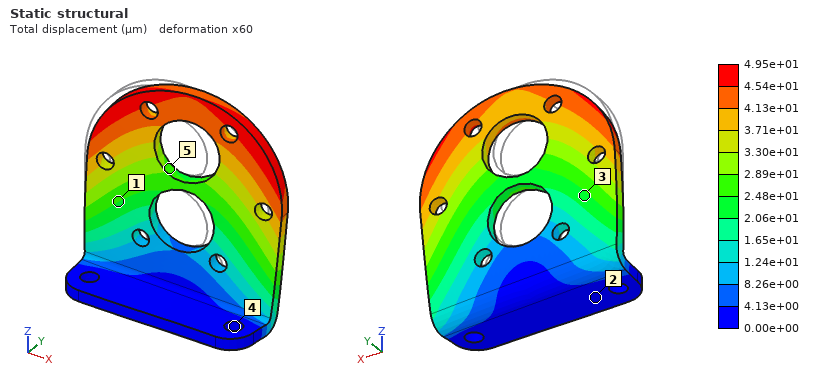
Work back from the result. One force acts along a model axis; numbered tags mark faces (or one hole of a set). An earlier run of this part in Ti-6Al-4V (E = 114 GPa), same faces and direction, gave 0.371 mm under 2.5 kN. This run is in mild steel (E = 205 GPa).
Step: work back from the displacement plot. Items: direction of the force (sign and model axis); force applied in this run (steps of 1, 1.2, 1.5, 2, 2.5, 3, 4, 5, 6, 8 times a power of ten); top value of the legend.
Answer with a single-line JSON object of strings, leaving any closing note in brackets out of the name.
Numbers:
{"direction of the force": "+X", "force applied in this run": "600 N", "top value of the legend": "4.95e+01 µm"}
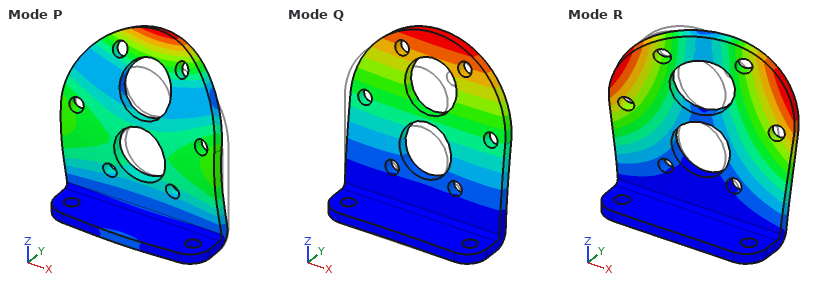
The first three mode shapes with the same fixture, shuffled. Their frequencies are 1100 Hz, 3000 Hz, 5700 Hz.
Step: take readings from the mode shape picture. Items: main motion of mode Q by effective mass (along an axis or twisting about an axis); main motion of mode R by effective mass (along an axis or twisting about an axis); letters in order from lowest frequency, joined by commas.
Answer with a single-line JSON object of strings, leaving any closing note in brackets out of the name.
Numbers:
{"main motion of mode Q by effective mass": "along Y", "main motion of mode R by effective mass": "twisting about Z", "letters in order from lowest frequency, joined by commas": "Q, R, P"}
